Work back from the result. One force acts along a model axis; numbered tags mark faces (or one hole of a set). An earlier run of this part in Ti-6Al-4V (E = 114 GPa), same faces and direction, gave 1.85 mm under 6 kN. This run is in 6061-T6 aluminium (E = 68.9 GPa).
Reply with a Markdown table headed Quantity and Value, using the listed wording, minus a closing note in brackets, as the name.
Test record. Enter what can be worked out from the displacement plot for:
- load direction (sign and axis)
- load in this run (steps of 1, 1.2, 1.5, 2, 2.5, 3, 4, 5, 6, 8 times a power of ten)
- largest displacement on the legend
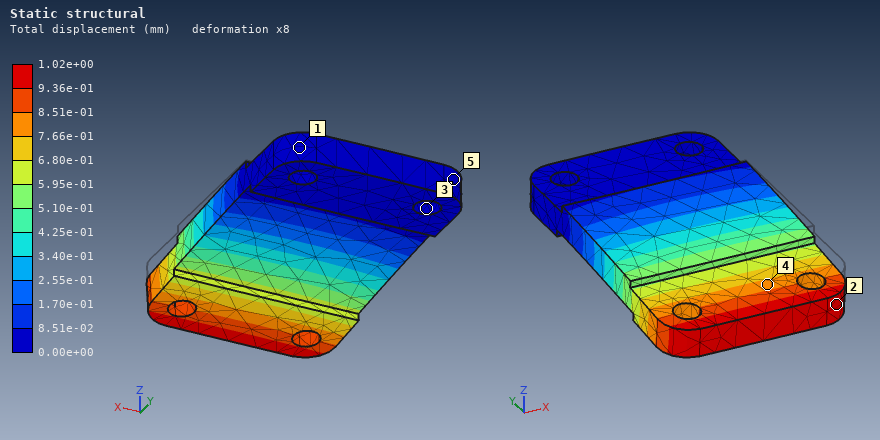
| Quantity | Value |
|---|---|
| load direction | -Z |
| load in this run | 2 kN |
| largest displacement on the legend | 1.02e+00 mm |
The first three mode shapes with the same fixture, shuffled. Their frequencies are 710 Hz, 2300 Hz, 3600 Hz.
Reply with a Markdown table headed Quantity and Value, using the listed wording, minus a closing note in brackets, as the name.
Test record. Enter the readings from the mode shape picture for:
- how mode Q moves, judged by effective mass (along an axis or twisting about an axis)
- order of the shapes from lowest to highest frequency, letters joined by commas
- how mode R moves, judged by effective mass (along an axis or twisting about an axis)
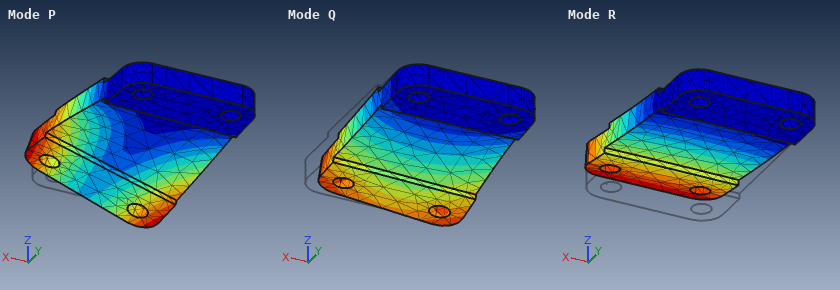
| Quantity | Value |
|---|---|
| how mode Q moves, judged by effective mass | along X |
| order of the shapes from lowest to highest frequency, letters joined by commas | R, P, Q |
| how mode R moves, judged by effective mass | along Z |
